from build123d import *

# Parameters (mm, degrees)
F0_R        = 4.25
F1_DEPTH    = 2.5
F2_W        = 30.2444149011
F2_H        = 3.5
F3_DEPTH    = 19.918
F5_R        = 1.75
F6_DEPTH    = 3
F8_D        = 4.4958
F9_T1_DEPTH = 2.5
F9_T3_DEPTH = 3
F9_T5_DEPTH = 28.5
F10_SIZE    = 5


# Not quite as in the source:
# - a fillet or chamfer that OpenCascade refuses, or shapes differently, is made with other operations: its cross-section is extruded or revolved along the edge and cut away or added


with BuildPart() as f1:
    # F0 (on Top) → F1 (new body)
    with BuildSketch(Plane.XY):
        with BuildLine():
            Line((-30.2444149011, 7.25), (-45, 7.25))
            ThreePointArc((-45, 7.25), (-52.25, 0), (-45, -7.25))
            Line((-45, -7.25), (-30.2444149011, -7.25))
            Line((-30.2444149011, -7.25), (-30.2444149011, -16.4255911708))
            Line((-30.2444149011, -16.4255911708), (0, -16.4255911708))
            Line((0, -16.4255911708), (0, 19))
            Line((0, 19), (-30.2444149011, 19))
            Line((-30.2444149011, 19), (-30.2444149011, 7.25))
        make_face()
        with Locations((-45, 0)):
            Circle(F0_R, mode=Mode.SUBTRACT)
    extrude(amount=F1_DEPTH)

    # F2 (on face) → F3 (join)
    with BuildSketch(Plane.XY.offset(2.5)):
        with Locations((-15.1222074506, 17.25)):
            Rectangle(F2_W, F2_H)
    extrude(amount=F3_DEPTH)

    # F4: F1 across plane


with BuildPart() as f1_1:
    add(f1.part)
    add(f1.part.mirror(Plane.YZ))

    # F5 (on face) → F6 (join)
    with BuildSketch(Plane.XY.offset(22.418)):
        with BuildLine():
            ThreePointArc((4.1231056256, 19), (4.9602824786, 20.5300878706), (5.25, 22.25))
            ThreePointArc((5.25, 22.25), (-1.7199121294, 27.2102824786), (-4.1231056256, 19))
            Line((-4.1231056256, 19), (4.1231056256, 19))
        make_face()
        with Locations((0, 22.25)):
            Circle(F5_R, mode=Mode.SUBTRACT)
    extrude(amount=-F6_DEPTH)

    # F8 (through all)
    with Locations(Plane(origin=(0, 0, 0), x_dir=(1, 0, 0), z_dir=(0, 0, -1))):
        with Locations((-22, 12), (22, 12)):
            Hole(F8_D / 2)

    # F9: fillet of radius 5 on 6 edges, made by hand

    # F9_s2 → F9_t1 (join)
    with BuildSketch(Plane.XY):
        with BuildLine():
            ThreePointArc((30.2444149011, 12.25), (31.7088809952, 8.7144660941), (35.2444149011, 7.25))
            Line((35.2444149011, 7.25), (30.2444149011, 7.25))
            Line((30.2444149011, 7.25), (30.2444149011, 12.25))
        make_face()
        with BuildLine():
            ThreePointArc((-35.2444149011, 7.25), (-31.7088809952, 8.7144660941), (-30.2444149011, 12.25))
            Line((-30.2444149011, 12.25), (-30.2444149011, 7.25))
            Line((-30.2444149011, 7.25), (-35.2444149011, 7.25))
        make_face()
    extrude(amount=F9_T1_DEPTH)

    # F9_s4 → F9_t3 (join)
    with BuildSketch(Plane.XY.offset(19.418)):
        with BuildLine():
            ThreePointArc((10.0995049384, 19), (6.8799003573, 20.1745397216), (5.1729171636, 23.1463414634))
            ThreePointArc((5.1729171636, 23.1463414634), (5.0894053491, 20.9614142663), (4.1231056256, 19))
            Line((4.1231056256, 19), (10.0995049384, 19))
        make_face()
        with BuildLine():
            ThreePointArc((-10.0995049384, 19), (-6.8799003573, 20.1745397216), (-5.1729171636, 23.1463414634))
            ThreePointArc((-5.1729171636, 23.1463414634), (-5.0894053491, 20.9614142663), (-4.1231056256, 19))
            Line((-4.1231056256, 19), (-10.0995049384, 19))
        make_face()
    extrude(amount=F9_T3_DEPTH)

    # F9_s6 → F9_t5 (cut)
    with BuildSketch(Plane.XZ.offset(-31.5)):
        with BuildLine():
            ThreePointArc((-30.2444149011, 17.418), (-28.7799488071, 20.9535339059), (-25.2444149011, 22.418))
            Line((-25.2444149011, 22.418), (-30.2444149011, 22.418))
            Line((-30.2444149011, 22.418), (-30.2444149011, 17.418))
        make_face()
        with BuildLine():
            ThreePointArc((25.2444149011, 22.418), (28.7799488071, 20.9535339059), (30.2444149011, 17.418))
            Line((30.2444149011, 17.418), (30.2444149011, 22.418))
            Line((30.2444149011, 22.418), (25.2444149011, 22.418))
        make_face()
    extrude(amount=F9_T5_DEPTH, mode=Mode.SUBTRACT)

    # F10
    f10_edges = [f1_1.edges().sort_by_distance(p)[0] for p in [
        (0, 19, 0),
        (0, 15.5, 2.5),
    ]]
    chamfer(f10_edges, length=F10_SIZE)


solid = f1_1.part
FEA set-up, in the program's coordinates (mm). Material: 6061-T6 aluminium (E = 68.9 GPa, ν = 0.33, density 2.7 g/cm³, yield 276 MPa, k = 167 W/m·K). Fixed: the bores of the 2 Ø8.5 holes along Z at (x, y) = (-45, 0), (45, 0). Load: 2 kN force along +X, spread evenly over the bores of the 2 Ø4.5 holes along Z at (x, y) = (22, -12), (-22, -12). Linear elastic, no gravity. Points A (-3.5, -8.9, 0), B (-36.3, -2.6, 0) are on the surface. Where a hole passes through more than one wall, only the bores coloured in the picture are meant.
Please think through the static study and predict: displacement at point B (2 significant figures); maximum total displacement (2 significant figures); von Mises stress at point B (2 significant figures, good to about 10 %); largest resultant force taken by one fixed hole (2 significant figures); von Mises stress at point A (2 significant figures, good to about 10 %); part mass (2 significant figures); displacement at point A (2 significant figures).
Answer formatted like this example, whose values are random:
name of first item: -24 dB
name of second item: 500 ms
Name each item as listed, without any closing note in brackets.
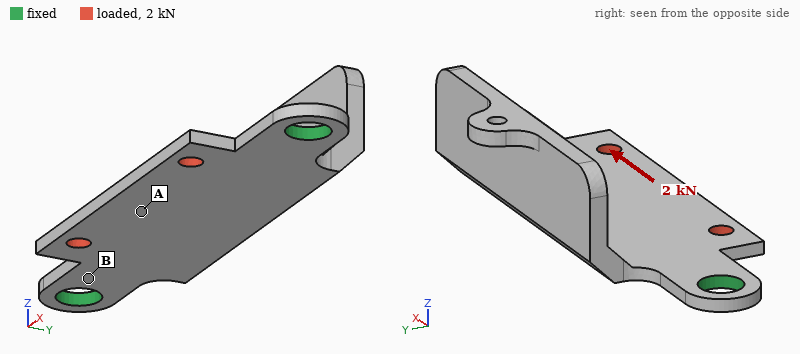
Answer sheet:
displacement at point B: 3.3 µm
maximum total displacement: 21 µm
von Mises stress at point B: 42 MPa
largest resultant force taken by one fixed hole: 1.0 kN
von Mises stress at point A: 11 MPa
part mass: 29 g
displacement at point A: 12 µm
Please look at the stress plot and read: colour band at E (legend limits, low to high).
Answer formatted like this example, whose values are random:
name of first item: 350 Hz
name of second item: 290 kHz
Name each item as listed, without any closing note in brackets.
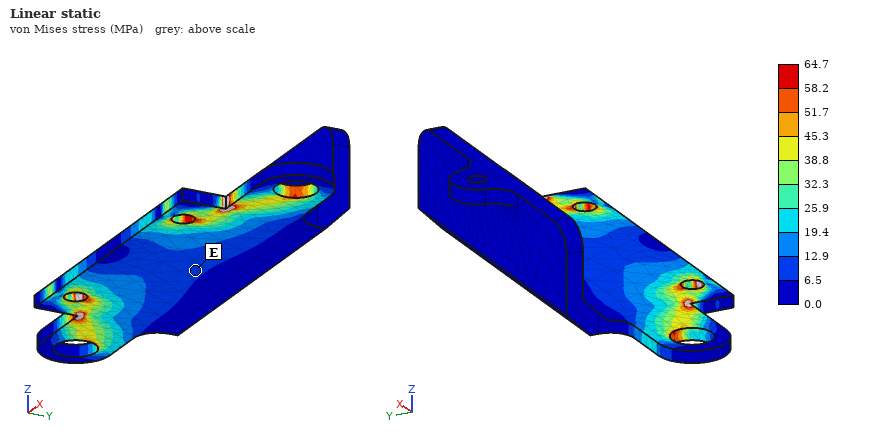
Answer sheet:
colour band at E: 6.5 to 12.9 MPa
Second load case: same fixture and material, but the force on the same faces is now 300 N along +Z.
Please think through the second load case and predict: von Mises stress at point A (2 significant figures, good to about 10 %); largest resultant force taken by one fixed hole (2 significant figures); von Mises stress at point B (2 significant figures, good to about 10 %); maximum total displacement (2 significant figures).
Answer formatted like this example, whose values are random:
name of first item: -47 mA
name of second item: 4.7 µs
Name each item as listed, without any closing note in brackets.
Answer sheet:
von Mises stress at point A: 14 MPa
largest resultant force taken by one fixed hole: 150 N
von Mises stress at point B: 110 MPa
maximum total displacement: 0.43 mm
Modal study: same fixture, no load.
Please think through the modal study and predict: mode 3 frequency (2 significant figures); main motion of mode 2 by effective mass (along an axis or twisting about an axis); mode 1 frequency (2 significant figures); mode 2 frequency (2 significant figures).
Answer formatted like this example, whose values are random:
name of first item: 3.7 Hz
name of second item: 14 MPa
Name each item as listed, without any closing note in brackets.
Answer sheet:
mode 3 frequency: 3000 Hz
main motion of mode 2 by effective mass: along Z
mode 1 frequency: 970 Hz
mode 2 frequency: 2000 Hz
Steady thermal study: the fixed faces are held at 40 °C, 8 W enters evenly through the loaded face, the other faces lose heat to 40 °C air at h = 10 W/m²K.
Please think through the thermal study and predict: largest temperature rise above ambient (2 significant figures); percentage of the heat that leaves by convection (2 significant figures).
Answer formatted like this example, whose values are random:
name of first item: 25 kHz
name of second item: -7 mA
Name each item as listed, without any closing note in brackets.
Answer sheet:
largest temperature rise above ambient: 15 K
percentage of the heat that leaves by convection: 8.8 %
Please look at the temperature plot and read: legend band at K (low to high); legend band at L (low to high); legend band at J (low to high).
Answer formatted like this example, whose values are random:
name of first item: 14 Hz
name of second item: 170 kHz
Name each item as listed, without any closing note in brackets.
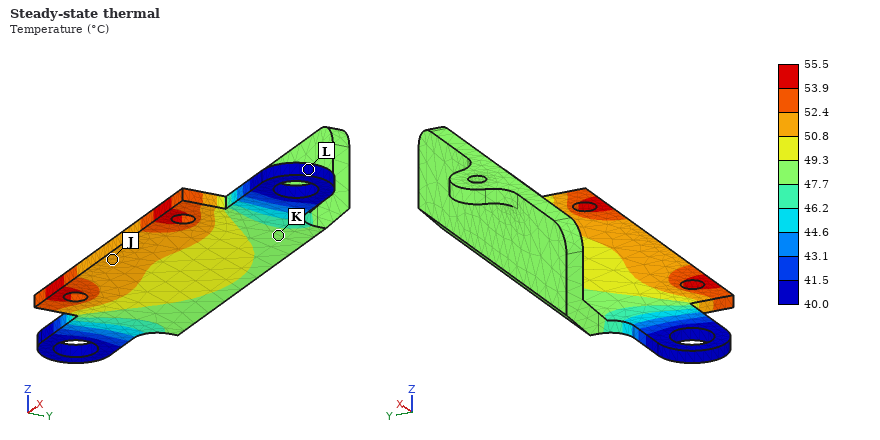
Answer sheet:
legend band at K: 47.7 to 49.3 °C
legend band at L: 40.0 to 41.5 °C
legend band at J: 50.8 to 52.4 °C
